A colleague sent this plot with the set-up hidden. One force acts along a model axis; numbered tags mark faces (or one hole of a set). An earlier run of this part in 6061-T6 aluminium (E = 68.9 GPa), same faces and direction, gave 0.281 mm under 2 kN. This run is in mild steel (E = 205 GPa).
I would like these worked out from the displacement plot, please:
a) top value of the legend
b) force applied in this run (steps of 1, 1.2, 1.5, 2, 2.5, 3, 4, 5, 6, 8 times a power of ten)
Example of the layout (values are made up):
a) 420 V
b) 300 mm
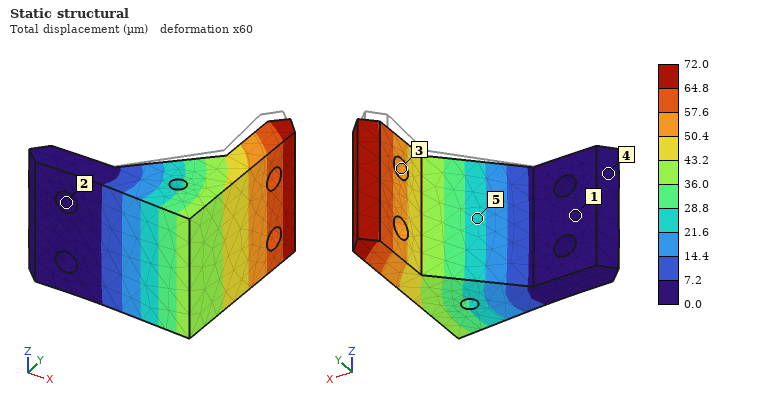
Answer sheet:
a) 72.0 µm
b) 1.5 kN
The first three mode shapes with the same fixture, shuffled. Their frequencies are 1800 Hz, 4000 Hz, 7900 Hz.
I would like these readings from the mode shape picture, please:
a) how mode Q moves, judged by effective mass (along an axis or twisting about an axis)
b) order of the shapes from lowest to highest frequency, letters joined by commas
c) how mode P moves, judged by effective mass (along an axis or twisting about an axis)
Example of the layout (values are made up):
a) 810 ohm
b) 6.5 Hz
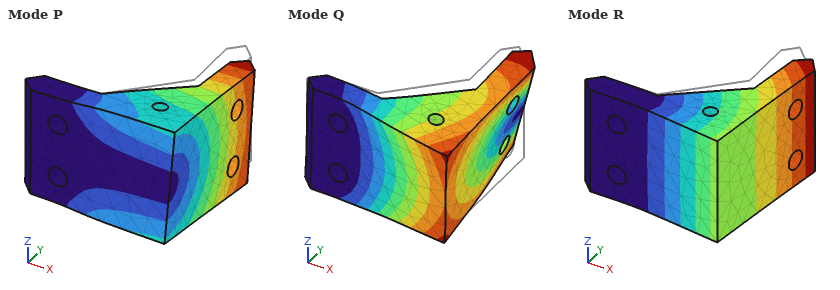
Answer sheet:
a) along Z
b) R, P, Q
c) along Z
